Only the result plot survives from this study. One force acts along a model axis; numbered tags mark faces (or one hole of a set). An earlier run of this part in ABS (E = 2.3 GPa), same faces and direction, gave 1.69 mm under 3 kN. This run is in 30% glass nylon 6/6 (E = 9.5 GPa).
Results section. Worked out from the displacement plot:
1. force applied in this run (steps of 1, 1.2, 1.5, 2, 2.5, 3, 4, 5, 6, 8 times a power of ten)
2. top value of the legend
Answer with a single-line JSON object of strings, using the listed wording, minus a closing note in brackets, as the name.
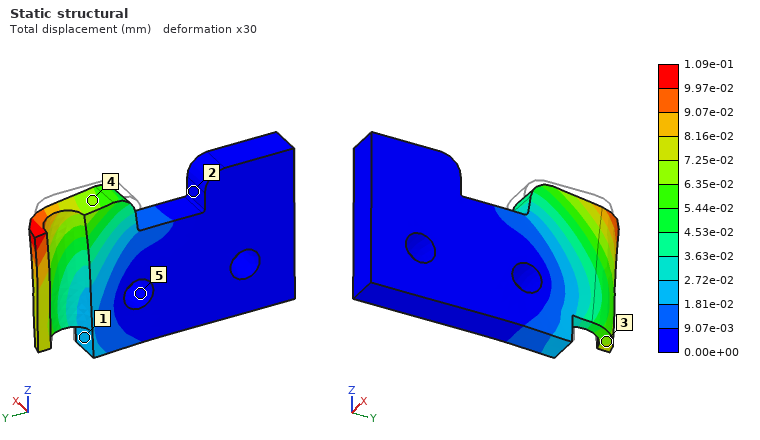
{"force applied in this run": "800 N", "top value of the legend": "1.09e-01 mm"}
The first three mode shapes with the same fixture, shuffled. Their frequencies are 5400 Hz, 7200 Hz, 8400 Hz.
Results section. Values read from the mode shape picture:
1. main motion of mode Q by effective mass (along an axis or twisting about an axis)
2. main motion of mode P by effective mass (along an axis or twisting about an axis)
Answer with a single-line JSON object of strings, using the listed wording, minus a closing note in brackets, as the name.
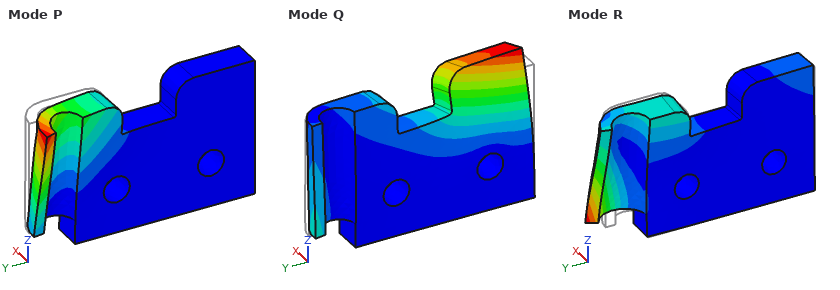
{"main motion of mode Q by effective mass": "along X", "main motion of mode P by effective mass": "along X"}
